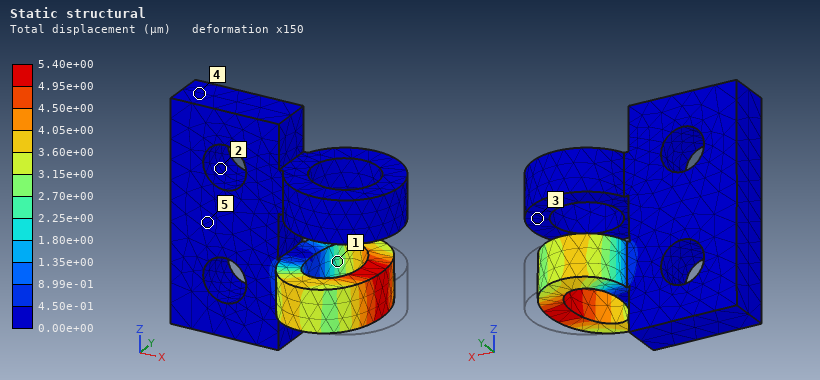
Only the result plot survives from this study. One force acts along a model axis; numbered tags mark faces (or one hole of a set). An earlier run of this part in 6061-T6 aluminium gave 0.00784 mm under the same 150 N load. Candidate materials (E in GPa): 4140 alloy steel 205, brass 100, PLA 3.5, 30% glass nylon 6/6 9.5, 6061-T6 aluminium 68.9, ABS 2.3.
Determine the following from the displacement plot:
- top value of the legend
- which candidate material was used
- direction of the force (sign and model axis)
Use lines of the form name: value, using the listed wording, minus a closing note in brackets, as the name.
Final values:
top value of the legend: 5.40e+00 µm
which candidate material was used: brass
direction of the force: -X
